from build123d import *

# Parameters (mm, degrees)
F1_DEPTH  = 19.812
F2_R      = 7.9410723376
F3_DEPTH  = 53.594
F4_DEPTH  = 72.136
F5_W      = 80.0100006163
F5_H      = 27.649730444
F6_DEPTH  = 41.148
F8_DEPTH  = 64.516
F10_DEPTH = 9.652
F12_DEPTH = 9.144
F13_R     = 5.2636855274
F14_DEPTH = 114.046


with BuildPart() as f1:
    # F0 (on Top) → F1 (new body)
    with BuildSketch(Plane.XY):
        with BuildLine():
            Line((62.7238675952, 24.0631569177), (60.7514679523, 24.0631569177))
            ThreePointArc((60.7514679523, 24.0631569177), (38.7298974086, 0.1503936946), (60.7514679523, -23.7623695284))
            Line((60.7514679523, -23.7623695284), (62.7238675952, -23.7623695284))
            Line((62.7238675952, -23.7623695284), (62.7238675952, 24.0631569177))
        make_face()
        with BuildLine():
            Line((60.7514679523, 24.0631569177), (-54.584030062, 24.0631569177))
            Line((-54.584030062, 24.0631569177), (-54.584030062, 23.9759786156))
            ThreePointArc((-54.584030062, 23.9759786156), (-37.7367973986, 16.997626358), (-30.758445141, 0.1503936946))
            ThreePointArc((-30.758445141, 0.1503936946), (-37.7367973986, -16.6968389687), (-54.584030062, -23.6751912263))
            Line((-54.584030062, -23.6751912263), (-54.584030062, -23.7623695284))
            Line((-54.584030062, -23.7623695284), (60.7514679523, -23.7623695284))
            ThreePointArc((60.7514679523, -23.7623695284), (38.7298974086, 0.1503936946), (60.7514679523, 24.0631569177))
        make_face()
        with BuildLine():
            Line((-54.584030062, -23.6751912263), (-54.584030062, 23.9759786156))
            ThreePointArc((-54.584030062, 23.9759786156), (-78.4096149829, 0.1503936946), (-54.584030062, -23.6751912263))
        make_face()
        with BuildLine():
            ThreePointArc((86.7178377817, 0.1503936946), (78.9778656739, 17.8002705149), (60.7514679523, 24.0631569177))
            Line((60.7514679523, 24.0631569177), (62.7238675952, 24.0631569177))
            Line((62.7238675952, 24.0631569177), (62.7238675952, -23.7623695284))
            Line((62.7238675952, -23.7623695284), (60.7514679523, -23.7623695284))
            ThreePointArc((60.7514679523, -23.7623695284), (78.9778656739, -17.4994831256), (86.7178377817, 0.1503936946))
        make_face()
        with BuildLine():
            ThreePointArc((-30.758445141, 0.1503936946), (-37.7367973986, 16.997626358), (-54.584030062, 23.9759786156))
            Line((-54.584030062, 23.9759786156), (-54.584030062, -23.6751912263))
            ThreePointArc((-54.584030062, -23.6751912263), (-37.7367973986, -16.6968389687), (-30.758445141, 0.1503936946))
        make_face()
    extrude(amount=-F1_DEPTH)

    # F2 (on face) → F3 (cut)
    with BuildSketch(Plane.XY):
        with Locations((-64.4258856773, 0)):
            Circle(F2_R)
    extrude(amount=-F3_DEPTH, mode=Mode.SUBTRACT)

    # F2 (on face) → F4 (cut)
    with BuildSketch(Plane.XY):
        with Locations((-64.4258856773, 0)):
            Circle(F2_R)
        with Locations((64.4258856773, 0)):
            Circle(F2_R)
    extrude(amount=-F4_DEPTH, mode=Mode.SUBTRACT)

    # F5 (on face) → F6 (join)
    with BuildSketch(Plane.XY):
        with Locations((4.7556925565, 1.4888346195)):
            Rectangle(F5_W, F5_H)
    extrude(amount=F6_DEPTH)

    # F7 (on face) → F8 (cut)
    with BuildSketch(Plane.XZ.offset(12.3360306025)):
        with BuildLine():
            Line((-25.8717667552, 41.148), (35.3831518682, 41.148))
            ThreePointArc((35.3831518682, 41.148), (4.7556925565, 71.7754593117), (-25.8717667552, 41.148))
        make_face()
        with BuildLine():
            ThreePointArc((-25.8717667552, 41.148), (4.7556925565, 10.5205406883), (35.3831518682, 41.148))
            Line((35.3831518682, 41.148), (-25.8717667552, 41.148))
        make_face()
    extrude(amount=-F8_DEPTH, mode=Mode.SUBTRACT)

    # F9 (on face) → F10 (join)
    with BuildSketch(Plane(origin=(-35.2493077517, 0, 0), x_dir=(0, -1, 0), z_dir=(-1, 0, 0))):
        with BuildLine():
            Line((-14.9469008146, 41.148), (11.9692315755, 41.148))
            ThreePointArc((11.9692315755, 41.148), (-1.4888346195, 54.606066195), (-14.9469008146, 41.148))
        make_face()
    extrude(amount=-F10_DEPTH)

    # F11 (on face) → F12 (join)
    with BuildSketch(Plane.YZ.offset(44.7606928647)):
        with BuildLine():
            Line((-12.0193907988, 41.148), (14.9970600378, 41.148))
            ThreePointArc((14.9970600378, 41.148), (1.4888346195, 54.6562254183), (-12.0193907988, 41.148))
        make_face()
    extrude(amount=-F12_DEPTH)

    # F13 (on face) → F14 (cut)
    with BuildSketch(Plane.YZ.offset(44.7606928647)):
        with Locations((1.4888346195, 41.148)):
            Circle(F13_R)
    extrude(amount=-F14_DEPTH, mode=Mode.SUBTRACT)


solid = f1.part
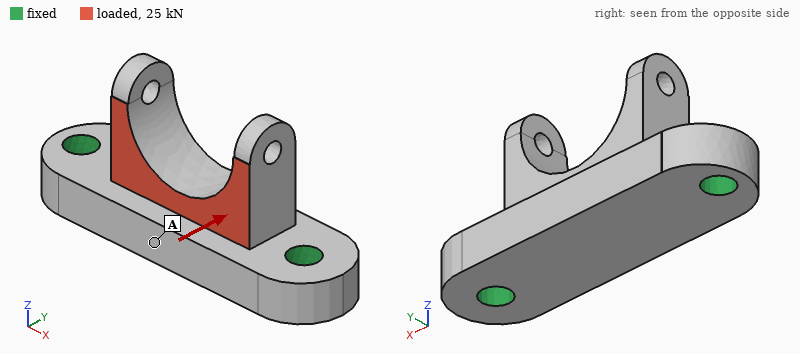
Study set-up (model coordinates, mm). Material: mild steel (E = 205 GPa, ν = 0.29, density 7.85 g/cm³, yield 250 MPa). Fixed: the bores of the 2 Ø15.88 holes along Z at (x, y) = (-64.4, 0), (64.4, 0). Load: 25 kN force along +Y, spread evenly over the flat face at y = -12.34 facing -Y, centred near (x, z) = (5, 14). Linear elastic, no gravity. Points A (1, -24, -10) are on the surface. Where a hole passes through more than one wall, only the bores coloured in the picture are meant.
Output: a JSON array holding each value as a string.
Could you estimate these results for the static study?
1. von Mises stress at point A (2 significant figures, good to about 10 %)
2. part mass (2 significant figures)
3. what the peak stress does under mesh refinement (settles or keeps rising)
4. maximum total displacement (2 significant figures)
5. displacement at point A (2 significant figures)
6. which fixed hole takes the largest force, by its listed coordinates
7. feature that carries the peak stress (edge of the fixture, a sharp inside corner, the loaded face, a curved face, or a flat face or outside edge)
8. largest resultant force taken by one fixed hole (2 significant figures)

["29 MPa", "1.5 kg", "keeps rising", "0.10 mm", "0.030 mm", "(64.4, 0)", "edge of the fixture", "14 kN"]
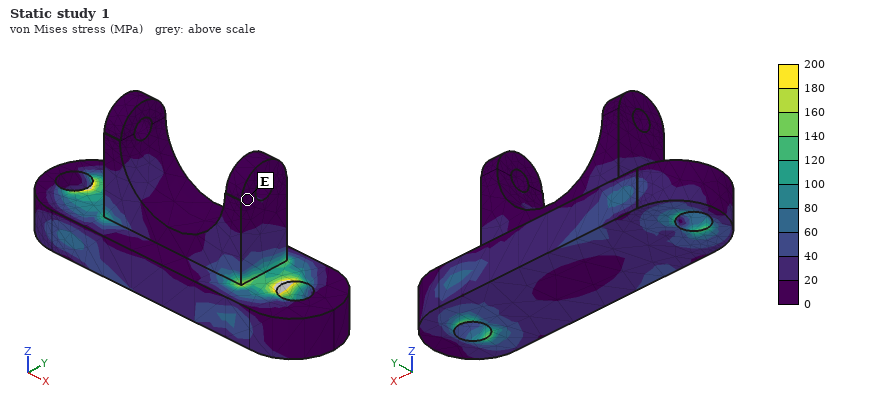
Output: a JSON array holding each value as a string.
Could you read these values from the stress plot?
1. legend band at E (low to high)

["0 to 20 MPa"]
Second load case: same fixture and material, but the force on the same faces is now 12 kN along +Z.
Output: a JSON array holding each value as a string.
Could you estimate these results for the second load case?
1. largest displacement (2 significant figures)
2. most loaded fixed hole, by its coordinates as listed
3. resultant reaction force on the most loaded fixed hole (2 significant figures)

["28 µm", "(64.4, 0)", "6.8 kN"]
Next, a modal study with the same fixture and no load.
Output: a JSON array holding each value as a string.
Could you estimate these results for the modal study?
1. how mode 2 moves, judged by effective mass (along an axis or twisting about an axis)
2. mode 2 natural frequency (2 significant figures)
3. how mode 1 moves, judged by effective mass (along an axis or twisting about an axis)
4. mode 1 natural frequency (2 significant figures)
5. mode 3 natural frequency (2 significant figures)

["along Z", "5500 Hz", "along Y", "4400 Hz", "7300 Hz"]
